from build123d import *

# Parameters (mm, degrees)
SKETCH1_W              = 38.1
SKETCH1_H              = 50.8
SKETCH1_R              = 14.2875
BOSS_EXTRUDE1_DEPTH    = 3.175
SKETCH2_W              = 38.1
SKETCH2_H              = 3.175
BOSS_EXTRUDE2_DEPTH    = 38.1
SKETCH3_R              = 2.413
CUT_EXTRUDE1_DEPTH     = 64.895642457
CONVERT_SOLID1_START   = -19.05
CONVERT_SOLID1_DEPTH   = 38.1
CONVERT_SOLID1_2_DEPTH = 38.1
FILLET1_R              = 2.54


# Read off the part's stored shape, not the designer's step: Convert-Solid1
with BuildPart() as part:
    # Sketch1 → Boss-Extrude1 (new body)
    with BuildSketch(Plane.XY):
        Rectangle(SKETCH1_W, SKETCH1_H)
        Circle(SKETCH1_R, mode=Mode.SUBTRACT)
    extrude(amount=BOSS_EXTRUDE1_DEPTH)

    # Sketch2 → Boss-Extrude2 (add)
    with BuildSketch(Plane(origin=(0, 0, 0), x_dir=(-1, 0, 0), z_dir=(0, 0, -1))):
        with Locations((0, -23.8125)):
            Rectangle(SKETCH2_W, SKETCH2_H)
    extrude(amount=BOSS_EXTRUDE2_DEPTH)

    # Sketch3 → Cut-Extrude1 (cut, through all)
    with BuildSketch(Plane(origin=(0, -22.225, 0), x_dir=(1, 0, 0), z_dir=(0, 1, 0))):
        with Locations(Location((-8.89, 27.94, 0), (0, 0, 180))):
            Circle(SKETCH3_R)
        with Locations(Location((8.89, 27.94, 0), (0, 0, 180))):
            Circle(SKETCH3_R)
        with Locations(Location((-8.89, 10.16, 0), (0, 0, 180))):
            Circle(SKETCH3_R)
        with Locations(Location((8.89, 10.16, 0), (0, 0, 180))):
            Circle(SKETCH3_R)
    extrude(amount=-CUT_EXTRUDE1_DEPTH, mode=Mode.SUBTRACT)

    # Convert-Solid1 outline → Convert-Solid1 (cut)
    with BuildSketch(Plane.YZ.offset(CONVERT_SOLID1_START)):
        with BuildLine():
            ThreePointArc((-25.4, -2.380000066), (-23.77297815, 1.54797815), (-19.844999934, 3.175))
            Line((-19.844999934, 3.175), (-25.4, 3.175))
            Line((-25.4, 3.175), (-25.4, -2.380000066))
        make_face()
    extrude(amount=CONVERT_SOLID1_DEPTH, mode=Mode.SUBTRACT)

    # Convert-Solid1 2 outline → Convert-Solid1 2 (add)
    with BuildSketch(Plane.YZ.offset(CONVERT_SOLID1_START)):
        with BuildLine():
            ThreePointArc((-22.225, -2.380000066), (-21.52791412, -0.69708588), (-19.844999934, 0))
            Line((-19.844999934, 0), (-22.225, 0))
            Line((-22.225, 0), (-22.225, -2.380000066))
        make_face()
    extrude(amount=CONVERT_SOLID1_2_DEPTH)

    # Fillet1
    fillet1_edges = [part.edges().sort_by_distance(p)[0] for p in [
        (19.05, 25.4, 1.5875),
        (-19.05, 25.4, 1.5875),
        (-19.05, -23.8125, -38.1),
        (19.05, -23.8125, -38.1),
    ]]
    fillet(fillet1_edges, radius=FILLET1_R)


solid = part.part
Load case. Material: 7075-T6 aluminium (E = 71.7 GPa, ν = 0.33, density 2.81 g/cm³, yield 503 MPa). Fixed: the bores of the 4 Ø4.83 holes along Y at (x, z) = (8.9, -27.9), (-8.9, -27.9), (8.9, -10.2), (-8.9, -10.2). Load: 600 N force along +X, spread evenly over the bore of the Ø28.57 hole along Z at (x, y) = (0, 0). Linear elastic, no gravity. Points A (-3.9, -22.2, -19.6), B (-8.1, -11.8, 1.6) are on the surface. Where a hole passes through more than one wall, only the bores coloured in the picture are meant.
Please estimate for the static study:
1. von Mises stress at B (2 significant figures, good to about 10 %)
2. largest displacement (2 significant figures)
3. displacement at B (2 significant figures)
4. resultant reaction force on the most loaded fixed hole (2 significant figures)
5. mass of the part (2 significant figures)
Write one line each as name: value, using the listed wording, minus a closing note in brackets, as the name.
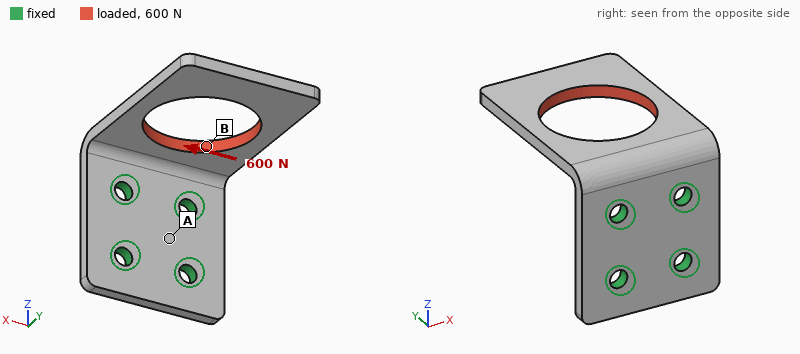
von Mises stress at B: 59 MPa
largest displacement: 0.30 mm
displacement at B: 0.070 mm
resultant reaction force on the most loaded fixed hole: 780 N
mass of the part: 23 g
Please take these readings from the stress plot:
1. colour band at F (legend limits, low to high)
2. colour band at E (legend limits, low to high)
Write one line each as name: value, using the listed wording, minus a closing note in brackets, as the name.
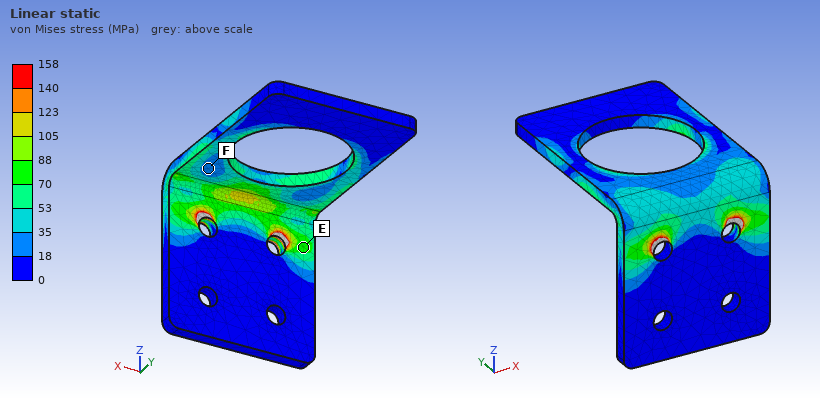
colour band at F: 18 to 35 MPa
colour band at E: 70 to 88 MPa
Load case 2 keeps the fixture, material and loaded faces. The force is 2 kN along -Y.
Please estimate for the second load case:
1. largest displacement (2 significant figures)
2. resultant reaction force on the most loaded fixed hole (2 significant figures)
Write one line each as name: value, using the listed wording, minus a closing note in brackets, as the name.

largest displacement: 0.81 mm
resultant reaction force on the most loaded fixed hole: 1.1 kN
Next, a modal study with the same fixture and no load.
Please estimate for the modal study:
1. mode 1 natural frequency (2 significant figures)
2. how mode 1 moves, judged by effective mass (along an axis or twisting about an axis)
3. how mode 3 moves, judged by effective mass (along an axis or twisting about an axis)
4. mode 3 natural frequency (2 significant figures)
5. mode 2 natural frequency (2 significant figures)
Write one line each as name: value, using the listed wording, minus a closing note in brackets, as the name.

mode 1 natural frequency: 740 Hz
how mode 1 moves, judged by effective mass: along Z
how mode 3 moves, judged by effective mass: along X
mode 3 natural frequency: 2700 Hz
mode 2 natural frequency: 2000 Hz
